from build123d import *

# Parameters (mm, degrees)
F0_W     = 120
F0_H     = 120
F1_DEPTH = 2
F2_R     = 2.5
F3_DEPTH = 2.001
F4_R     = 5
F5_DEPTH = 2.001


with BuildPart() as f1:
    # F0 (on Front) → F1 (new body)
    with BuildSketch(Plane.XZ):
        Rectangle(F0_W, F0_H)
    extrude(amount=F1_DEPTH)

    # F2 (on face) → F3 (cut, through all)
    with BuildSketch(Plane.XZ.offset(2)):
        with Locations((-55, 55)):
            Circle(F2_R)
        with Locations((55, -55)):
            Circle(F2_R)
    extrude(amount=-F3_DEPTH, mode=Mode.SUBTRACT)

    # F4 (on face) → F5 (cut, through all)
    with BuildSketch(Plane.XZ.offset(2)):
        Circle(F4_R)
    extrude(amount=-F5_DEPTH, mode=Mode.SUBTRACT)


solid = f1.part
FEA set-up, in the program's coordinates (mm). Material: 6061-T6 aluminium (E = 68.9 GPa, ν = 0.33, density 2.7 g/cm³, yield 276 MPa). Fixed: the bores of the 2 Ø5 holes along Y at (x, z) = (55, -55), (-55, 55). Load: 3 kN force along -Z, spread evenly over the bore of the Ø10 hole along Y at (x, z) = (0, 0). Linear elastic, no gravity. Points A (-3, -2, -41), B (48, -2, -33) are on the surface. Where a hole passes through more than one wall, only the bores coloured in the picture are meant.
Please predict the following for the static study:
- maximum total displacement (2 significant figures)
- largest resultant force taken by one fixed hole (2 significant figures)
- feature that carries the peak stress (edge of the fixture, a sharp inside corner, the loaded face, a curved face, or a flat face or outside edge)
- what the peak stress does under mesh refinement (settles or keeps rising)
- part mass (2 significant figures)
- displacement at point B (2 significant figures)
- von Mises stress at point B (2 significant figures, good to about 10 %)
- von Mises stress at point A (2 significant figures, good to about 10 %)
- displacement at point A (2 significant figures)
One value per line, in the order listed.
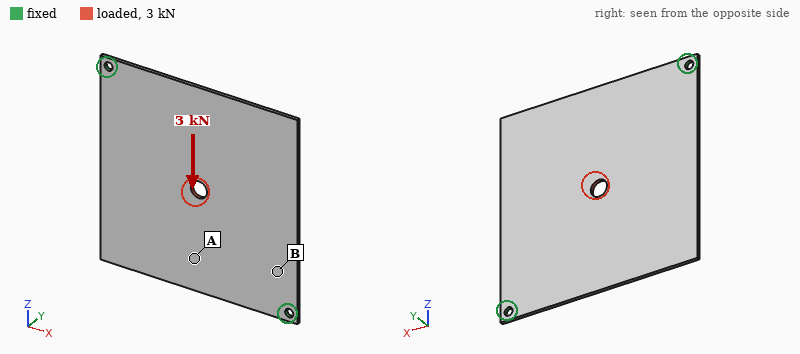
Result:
52 µm
1.5 kN
edge of the fixture
keeps rising
77 g
23 µm
28 MPa
12 MPa
42 µm
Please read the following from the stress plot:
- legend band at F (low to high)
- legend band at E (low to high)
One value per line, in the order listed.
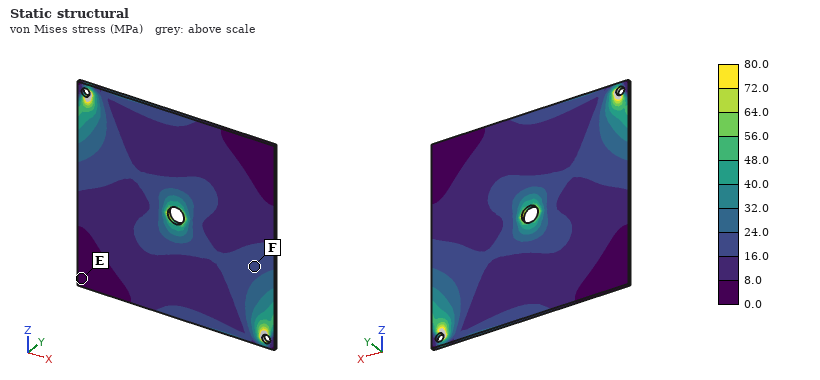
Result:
16.0 to 24.0 MPa
0.0 to 8.0 MPa
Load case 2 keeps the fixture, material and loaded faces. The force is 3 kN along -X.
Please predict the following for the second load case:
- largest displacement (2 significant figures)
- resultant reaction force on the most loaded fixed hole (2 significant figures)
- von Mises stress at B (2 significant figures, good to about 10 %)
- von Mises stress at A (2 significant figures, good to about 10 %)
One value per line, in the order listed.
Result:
52 µm
1.5 kN
11 MPa
15 MPa
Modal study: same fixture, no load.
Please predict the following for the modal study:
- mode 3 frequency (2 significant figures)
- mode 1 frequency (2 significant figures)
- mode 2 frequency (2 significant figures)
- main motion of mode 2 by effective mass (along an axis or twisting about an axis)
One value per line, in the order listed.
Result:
720 Hz
180 Hz
240 Hz
along Y
